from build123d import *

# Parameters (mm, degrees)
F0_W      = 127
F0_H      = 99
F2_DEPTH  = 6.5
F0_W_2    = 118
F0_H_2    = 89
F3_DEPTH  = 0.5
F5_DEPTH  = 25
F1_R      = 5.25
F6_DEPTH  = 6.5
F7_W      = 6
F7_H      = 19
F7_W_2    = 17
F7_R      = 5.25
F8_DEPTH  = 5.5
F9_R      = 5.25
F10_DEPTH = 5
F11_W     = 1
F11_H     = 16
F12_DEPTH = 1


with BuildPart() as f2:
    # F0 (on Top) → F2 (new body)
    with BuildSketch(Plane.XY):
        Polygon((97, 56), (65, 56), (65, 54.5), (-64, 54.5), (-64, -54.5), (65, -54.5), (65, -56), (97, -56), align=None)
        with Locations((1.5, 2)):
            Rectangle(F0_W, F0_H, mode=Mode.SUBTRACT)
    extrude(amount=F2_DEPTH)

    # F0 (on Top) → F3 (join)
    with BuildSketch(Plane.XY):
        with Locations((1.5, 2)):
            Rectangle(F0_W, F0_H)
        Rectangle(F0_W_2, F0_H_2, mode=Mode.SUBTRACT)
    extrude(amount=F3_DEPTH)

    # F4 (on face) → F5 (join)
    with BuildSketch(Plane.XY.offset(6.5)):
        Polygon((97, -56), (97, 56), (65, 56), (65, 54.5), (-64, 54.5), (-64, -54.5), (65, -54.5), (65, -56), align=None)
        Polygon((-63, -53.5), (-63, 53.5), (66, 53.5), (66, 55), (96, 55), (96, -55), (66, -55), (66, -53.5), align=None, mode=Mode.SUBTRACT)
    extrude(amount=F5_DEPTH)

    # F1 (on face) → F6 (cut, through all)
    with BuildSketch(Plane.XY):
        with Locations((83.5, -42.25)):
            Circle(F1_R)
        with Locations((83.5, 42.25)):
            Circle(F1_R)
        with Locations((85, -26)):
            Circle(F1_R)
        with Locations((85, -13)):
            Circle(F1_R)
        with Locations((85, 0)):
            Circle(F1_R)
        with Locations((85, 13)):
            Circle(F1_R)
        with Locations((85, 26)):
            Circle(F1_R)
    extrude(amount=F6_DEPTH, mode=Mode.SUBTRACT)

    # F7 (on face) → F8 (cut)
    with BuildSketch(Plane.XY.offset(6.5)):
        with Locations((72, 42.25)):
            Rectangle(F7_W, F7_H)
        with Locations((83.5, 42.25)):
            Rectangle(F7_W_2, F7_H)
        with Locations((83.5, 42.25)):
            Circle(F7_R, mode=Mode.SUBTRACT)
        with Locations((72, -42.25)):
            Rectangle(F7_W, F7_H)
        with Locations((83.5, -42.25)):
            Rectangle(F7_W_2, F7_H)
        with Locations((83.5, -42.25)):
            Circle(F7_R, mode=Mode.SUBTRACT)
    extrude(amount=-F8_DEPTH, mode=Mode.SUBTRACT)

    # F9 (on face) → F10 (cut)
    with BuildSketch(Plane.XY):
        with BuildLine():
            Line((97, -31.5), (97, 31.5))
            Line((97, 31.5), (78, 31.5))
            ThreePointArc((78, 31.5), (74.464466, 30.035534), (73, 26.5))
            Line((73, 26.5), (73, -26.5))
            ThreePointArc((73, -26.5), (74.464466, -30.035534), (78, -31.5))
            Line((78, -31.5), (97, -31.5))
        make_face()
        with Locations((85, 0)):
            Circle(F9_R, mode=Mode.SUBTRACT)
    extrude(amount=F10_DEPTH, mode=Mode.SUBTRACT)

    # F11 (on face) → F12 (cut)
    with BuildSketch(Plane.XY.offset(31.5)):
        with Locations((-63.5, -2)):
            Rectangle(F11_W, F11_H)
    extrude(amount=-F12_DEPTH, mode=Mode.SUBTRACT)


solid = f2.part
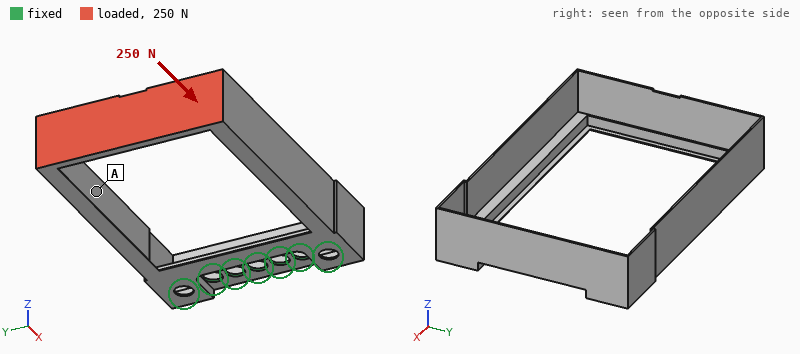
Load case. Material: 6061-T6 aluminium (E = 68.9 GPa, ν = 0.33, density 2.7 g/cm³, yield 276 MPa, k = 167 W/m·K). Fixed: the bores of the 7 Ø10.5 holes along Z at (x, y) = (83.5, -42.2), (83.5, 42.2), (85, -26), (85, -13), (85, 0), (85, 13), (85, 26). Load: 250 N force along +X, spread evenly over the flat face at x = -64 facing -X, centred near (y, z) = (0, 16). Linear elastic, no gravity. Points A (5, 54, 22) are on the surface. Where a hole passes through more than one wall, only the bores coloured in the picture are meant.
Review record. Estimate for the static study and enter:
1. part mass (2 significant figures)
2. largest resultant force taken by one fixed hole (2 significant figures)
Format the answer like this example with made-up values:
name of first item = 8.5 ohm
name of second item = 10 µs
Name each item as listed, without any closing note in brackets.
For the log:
part mass = 93 g
largest resultant force taken by one fixed hole = 160 N
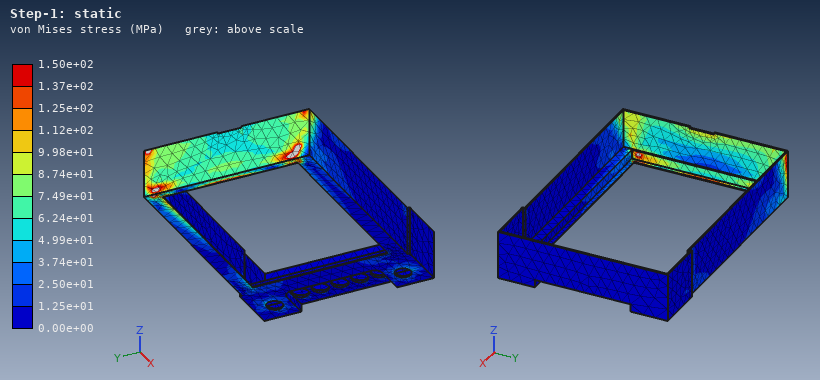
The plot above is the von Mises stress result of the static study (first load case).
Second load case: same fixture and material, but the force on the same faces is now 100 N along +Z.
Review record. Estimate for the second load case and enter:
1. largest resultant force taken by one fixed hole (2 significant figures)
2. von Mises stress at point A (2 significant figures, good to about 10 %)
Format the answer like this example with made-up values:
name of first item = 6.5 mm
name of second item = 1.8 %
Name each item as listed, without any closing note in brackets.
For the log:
largest resultant force taken by one fixed hole = 600 N
von Mises stress at point A = 11 MPa
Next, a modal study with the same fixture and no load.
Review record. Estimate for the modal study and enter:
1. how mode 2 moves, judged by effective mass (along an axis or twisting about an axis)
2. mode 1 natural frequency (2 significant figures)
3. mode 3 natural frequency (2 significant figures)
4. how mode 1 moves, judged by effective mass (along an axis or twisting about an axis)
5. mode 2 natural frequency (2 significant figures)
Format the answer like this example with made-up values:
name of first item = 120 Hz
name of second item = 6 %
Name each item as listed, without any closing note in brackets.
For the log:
how mode 2 moves, judged by effective mass = along Z
mode 1 natural frequency = 230 Hz
mode 3 natural frequency = 360 Hz
how mode 1 moves, judged by effective mass = along Y
mode 2 natural frequency = 270 Hz
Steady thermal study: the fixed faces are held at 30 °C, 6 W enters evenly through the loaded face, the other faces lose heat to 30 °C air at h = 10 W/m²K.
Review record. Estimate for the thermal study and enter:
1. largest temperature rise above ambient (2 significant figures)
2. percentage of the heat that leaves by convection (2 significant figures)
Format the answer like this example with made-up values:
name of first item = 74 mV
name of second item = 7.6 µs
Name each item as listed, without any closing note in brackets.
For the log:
largest temperature rise above ambient = 32 K
percentage of the heat that leaves by convection = 62 %
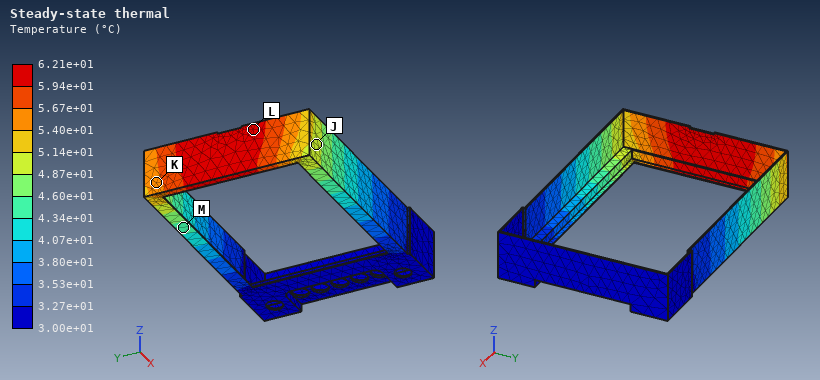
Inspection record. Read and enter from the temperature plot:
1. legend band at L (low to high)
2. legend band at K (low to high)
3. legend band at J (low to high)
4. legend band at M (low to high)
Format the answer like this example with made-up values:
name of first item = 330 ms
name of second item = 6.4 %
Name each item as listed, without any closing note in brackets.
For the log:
legend band at L = 5.94e+01 to 6.21e+01 °C
legend band at K = 5.40e+01 to 5.67e+01 °C
legend band at J = 4.87e+01 to 5.14e+01 °C
legend band at M = 4.34e+01 to 4.60e+01 °C
